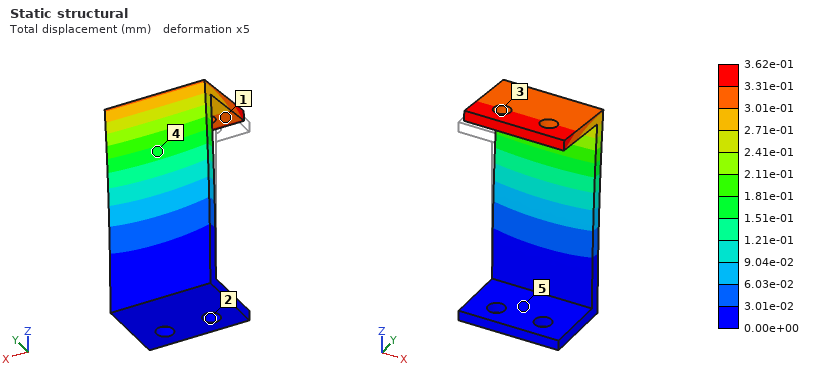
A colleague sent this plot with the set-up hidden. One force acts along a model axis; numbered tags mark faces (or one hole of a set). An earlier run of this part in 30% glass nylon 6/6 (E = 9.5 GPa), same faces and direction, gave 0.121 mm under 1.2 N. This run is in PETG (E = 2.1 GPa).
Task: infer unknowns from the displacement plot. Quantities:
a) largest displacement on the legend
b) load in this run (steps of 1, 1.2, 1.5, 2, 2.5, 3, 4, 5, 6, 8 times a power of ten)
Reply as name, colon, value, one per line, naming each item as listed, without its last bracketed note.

largest displacement on the legend: 3.62e-01 mm
load in this run: 0.8 N
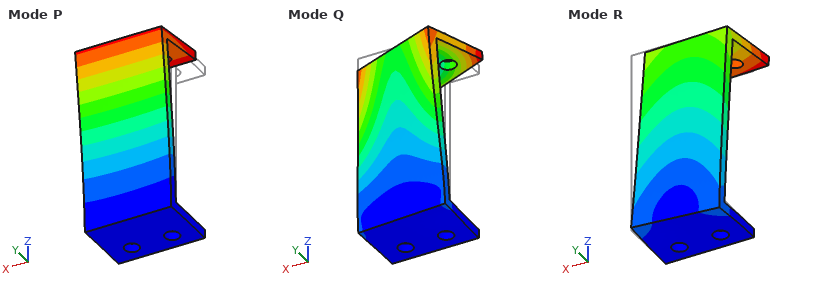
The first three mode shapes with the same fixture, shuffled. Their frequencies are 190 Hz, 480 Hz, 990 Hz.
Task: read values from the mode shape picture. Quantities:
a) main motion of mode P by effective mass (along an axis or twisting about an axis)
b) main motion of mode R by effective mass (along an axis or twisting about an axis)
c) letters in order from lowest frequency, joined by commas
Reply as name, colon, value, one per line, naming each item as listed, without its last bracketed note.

main motion of mode P by effective mass: along Y
main motion of mode R by effective mass: along X
letters in order from lowest frequency, joined by commas: P, R, Q
